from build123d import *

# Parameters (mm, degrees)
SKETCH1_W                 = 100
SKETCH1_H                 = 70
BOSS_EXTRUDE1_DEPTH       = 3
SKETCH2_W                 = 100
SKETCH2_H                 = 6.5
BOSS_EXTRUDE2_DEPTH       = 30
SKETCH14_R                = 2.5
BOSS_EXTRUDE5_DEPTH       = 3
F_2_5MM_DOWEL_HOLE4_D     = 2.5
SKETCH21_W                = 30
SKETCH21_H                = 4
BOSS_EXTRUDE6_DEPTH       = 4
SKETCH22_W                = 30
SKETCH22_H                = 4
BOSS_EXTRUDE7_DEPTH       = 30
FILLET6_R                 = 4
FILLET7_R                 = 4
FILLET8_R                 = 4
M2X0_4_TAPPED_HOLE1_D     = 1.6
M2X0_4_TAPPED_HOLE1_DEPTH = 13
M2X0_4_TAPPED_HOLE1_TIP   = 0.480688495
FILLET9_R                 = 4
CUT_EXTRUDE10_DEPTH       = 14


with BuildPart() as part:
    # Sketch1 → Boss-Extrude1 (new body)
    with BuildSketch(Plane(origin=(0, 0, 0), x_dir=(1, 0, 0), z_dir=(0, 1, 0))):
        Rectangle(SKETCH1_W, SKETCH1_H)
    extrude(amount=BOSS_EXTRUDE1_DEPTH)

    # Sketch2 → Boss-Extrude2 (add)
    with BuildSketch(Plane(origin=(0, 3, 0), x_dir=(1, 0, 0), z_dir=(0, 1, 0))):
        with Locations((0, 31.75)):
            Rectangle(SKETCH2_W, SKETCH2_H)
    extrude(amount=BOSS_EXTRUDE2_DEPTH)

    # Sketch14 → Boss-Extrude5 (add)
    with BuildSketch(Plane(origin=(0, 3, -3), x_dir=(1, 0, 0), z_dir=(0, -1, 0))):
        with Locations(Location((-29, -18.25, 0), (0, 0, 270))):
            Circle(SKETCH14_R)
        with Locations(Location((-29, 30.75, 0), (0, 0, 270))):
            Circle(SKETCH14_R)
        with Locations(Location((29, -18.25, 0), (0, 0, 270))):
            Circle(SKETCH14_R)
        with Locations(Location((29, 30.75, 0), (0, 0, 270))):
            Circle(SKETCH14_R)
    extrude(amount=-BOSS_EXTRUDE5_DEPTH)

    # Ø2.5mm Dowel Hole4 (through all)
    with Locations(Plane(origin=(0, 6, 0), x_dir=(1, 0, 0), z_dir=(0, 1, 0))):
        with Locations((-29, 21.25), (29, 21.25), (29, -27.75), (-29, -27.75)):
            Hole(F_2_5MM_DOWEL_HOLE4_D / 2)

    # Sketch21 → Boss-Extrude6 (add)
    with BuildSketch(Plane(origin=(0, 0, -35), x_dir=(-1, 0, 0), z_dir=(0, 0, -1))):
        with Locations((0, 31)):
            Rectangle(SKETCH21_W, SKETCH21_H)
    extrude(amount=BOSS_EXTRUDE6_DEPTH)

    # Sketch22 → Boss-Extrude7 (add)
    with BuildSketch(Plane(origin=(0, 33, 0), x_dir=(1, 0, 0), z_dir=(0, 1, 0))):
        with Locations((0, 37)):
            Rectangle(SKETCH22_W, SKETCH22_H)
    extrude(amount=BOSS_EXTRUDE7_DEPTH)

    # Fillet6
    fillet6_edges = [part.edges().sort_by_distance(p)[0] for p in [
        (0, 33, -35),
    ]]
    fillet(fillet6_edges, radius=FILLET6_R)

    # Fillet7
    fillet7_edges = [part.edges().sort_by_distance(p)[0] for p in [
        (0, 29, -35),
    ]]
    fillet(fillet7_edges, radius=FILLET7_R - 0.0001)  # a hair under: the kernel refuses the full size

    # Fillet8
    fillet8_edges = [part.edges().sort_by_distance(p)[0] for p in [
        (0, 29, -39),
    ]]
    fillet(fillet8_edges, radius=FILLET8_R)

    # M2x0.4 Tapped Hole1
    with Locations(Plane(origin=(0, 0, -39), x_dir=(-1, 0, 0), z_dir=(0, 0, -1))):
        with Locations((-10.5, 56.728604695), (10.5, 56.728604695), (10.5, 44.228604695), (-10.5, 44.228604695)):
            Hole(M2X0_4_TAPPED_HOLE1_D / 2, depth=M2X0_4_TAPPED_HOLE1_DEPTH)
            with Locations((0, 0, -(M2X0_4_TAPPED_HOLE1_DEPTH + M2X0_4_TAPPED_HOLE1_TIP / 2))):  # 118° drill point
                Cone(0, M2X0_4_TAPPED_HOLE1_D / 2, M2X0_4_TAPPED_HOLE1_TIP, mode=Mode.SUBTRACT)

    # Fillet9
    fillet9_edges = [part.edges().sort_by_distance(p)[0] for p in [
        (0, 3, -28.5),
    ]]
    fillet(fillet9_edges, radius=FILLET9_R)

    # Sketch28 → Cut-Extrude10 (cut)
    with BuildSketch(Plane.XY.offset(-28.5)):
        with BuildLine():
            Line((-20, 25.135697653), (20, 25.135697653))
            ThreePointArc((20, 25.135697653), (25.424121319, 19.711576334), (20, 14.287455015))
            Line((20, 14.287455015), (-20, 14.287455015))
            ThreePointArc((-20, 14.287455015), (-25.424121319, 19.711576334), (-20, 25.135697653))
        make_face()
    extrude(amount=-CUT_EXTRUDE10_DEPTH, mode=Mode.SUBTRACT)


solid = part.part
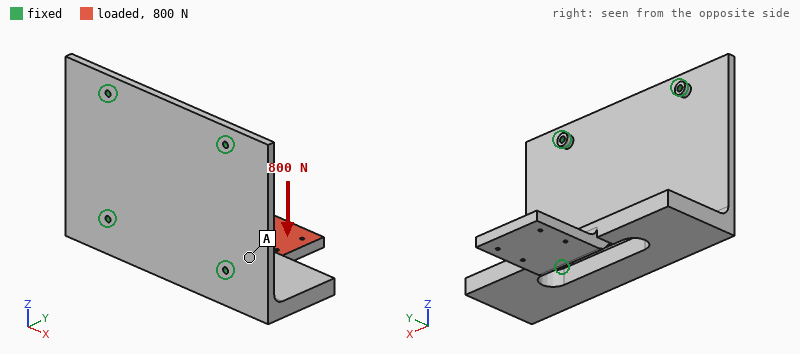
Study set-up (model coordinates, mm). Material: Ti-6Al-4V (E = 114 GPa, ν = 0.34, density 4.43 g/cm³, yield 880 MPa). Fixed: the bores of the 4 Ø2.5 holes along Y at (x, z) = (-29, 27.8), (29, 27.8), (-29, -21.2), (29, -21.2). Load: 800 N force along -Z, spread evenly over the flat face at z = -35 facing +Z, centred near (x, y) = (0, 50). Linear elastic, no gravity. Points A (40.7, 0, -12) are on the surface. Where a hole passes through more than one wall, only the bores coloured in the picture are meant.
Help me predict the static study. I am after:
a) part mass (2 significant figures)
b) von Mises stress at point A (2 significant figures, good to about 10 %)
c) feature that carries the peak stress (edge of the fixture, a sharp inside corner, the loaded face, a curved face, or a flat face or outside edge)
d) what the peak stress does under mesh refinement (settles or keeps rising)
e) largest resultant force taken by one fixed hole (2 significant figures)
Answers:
180 g
52 MPa
edge of the fixture
keeps rising
500 N
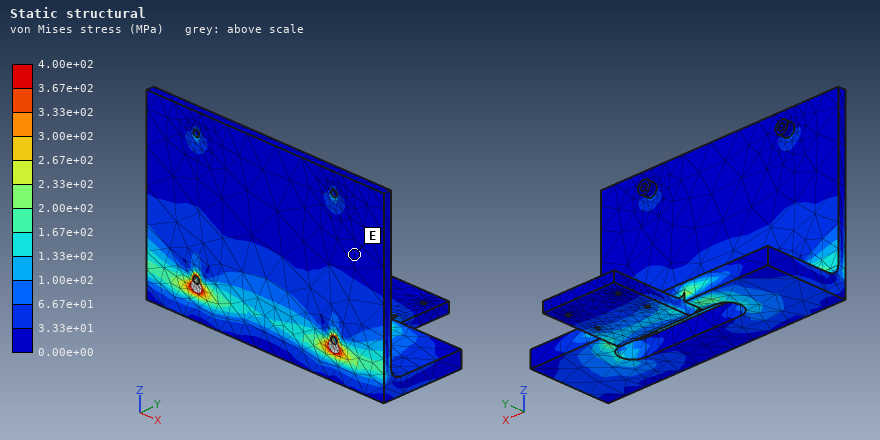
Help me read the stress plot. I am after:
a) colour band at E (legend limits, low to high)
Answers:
0.00e+00 to 3.33e+01 MPa
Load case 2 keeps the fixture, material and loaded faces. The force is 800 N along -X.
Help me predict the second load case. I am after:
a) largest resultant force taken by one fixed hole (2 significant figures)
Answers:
770 N
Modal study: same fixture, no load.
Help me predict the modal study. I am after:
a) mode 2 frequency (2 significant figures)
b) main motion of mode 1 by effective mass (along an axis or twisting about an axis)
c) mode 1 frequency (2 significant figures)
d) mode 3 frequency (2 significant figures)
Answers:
2600 Hz
along Z
860 Hz
3000 Hz
